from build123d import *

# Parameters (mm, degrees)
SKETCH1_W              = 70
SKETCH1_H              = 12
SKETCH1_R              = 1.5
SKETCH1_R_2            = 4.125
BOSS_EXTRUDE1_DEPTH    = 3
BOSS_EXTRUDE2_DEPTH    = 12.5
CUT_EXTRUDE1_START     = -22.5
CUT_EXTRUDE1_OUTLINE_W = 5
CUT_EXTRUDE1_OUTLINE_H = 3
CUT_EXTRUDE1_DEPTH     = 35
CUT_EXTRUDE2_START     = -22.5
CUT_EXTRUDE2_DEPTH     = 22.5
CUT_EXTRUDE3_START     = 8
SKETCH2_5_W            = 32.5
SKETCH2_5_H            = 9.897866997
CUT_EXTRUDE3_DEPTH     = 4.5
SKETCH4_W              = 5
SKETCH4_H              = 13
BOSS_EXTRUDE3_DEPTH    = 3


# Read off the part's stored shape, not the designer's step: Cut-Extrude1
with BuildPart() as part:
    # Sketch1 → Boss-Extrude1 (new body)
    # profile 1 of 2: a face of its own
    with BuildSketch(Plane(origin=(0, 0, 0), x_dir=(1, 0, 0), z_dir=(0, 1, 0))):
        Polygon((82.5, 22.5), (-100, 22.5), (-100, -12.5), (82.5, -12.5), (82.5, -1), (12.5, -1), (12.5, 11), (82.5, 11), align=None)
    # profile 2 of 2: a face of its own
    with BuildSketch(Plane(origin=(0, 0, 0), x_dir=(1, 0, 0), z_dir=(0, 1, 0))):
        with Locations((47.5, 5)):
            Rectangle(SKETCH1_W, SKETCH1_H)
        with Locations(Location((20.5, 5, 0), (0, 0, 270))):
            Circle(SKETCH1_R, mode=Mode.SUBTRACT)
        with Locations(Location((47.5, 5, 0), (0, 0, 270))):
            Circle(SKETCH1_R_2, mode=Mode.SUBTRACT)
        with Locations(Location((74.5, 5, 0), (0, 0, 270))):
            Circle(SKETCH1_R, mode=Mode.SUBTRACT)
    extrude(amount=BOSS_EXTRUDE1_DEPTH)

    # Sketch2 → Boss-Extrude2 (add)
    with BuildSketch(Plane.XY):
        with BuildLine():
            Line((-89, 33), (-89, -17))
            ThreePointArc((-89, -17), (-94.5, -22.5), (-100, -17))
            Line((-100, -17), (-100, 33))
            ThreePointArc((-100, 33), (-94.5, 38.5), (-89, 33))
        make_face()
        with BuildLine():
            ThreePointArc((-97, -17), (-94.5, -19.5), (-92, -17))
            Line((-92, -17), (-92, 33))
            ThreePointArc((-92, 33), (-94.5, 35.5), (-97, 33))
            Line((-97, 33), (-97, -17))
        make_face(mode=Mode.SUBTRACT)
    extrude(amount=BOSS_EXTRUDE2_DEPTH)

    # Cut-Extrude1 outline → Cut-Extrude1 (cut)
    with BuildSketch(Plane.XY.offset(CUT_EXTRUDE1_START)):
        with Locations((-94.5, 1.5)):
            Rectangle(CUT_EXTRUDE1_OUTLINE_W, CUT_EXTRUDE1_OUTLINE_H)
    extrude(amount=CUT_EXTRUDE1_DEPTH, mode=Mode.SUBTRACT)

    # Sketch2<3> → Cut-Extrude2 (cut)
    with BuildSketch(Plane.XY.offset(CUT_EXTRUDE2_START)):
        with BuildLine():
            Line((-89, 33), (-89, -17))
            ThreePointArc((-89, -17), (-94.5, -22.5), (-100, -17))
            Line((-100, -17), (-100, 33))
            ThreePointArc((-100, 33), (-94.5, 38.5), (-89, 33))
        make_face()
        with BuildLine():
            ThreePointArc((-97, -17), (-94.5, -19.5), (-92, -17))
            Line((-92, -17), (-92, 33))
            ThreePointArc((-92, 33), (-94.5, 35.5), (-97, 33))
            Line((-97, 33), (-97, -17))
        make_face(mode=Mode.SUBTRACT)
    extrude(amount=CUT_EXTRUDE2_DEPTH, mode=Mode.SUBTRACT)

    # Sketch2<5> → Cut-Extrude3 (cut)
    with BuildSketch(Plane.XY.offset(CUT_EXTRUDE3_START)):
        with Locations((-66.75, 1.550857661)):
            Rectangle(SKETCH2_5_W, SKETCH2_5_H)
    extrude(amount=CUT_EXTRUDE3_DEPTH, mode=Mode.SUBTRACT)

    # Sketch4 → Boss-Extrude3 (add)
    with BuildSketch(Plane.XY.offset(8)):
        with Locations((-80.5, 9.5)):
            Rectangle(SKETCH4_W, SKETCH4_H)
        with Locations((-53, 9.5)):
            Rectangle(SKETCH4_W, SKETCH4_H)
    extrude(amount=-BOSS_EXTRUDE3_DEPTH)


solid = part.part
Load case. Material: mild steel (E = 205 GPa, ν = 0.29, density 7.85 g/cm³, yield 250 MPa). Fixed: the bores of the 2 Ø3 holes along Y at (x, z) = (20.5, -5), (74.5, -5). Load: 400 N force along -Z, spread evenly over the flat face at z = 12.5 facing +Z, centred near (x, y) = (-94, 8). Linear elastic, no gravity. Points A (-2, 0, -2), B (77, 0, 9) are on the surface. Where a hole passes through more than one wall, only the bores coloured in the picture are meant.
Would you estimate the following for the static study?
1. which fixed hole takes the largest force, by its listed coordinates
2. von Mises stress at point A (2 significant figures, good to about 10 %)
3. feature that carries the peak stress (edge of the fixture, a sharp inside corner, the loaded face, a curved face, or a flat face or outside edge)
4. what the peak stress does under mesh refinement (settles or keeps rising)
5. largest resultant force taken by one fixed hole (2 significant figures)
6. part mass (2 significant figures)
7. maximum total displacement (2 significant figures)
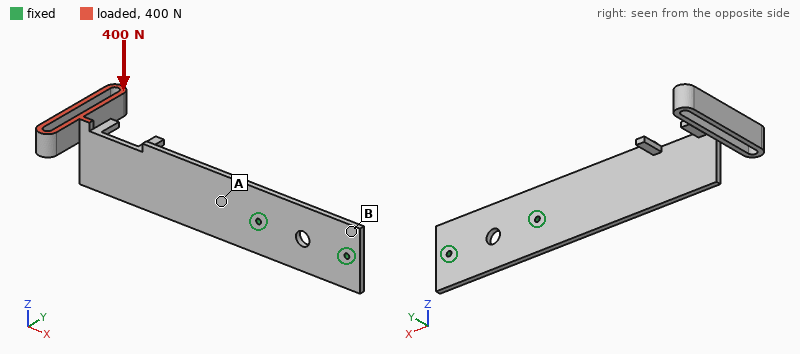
(20.5, -5)
35 MPa
edge of the fixture
keeps rising
1.2 kN
180 g
0.78 mm
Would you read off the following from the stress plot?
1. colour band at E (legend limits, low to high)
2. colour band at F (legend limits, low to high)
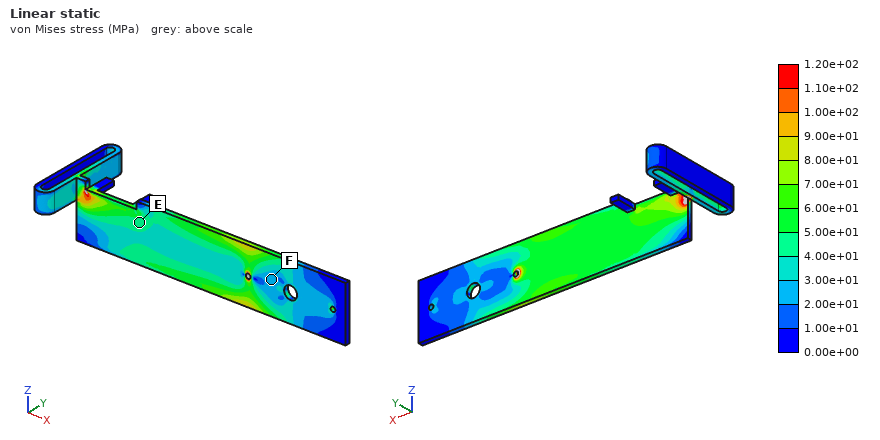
4.00e+01 to 5.00e+01 MPa
2.00e+01 to 3.00e+01 MPa
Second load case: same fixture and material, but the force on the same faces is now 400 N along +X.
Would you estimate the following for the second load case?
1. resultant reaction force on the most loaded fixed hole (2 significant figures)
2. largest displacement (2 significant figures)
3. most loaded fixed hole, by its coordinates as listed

350 N
1.5 mm
(20.5, -5)
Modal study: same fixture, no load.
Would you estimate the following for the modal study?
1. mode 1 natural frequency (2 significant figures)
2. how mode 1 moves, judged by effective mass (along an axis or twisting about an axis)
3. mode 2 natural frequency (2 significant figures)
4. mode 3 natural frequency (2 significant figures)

110 Hz
along Y
480 Hz
610 Hz
